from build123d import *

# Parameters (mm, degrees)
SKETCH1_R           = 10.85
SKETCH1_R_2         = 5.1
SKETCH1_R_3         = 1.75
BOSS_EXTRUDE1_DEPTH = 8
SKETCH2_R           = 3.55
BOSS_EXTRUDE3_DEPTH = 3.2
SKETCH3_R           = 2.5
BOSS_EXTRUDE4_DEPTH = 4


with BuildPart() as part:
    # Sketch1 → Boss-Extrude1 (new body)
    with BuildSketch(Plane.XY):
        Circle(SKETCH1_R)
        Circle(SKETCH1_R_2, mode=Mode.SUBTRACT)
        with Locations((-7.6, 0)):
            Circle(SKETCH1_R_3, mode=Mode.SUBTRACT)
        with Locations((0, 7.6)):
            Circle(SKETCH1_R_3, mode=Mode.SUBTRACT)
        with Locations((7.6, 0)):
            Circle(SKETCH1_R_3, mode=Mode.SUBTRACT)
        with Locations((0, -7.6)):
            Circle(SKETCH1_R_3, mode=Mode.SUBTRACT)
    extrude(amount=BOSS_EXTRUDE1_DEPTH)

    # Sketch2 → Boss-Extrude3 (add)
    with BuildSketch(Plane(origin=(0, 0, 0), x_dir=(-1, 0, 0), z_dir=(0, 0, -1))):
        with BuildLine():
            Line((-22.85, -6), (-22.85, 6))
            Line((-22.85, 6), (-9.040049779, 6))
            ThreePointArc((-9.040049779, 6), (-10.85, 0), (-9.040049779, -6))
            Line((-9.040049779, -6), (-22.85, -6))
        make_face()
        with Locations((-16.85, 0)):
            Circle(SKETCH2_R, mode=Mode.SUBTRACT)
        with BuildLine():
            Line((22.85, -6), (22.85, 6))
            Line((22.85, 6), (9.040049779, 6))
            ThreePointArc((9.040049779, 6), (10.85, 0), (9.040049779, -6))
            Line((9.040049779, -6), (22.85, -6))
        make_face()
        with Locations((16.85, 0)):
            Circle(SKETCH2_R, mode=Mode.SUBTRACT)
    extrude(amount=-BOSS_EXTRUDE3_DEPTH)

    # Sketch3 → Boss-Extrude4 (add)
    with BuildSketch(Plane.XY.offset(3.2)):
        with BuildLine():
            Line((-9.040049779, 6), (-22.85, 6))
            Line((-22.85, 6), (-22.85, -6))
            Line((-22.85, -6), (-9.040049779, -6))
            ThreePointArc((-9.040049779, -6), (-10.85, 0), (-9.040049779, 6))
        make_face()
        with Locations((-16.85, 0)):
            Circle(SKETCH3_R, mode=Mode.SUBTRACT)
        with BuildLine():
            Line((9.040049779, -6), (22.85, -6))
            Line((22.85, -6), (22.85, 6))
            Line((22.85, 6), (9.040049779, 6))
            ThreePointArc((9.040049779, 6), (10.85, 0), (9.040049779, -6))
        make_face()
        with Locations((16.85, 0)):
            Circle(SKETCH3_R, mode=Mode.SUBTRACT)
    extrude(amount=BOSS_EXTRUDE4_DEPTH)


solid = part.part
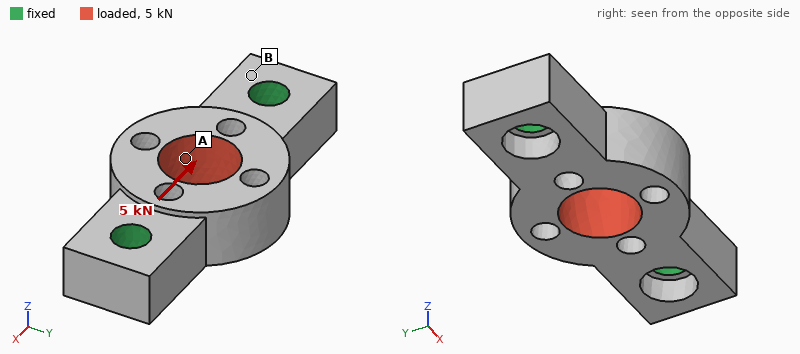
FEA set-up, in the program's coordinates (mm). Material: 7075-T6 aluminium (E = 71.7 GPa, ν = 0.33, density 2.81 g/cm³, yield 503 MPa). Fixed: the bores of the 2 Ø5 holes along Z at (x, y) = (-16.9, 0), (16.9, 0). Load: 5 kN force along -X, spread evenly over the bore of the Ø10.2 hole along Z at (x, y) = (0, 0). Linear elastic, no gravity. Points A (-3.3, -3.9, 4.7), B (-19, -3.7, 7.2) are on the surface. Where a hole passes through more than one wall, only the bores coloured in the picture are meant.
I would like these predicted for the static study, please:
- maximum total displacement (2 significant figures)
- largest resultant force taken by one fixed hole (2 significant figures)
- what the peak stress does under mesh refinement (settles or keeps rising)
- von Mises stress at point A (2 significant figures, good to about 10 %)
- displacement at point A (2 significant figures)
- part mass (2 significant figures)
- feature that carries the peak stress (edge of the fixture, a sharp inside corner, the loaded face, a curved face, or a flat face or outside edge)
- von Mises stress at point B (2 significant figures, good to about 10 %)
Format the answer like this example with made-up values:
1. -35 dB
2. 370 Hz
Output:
1. 9.2 µm
2. 2.5 kN
3. keeps rising
4. 37 MPa
5. 7.5 µm
6. 11 g
7. edge of the fixture
8. 14 MPa
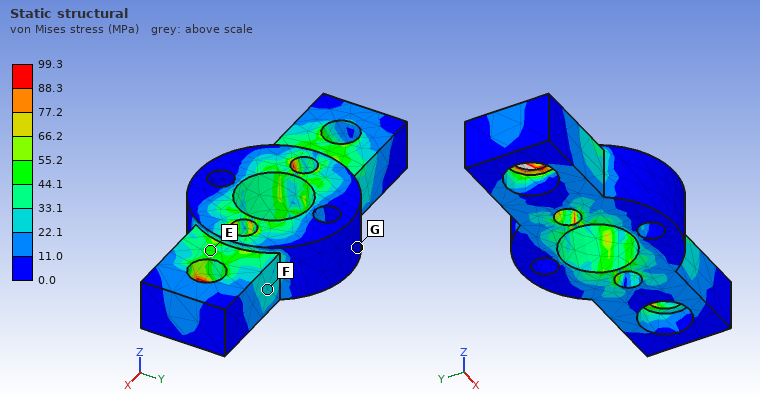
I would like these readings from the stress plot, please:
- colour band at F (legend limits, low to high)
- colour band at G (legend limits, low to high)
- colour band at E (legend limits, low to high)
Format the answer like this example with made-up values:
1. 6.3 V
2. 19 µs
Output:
1. 22.1 to 33.1 MPa
2. 0.0 to 11.0 MPa
3. 44.1 to 55.2 MPa
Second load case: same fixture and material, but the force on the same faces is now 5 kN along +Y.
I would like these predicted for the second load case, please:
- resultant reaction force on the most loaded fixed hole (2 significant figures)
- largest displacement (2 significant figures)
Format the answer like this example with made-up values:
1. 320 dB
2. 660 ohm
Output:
1. 2.5 kN
2. 34 µm
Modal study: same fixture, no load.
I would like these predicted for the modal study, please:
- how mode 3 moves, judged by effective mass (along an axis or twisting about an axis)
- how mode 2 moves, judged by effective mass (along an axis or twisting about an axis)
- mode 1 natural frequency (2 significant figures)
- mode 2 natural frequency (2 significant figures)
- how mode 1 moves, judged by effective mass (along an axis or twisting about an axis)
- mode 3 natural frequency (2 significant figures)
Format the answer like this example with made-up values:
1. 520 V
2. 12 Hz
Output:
1. along Y
2. along Z
3. 19 kHz
4. 19 kHz
5. twisting about X
6. 32 kHz
